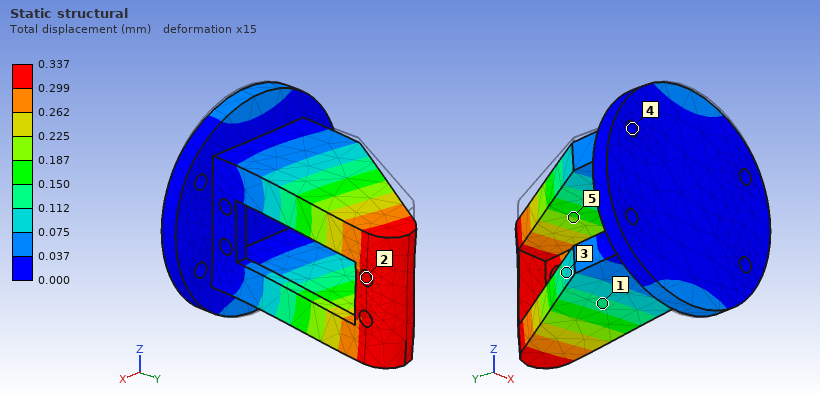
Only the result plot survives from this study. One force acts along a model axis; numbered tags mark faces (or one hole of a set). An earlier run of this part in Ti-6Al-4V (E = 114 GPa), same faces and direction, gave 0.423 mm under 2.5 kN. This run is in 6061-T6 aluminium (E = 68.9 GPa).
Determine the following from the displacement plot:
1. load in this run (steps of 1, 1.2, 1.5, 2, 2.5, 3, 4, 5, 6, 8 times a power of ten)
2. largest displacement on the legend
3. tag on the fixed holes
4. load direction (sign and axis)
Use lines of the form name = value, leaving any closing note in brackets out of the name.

load in this run = 1.2 kN
largest displacement on the legend = 0.337 mm
tag on the fixed holes = 4
load direction = -Z
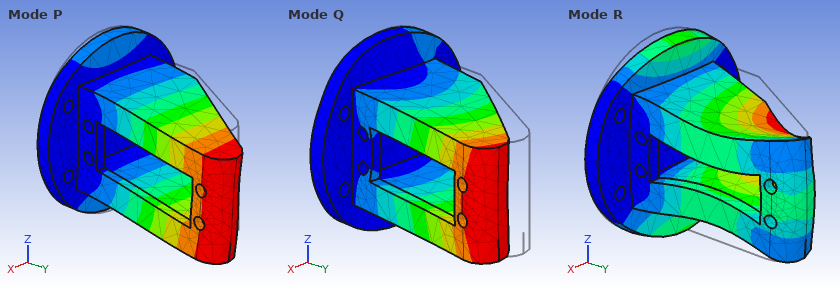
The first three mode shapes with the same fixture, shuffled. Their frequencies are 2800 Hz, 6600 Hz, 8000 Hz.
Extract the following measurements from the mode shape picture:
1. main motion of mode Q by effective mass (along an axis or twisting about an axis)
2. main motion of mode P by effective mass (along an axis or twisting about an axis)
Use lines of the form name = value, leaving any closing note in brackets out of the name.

main motion of mode Q by effective mass = along X
main motion of mode P by effective mass = along Z
